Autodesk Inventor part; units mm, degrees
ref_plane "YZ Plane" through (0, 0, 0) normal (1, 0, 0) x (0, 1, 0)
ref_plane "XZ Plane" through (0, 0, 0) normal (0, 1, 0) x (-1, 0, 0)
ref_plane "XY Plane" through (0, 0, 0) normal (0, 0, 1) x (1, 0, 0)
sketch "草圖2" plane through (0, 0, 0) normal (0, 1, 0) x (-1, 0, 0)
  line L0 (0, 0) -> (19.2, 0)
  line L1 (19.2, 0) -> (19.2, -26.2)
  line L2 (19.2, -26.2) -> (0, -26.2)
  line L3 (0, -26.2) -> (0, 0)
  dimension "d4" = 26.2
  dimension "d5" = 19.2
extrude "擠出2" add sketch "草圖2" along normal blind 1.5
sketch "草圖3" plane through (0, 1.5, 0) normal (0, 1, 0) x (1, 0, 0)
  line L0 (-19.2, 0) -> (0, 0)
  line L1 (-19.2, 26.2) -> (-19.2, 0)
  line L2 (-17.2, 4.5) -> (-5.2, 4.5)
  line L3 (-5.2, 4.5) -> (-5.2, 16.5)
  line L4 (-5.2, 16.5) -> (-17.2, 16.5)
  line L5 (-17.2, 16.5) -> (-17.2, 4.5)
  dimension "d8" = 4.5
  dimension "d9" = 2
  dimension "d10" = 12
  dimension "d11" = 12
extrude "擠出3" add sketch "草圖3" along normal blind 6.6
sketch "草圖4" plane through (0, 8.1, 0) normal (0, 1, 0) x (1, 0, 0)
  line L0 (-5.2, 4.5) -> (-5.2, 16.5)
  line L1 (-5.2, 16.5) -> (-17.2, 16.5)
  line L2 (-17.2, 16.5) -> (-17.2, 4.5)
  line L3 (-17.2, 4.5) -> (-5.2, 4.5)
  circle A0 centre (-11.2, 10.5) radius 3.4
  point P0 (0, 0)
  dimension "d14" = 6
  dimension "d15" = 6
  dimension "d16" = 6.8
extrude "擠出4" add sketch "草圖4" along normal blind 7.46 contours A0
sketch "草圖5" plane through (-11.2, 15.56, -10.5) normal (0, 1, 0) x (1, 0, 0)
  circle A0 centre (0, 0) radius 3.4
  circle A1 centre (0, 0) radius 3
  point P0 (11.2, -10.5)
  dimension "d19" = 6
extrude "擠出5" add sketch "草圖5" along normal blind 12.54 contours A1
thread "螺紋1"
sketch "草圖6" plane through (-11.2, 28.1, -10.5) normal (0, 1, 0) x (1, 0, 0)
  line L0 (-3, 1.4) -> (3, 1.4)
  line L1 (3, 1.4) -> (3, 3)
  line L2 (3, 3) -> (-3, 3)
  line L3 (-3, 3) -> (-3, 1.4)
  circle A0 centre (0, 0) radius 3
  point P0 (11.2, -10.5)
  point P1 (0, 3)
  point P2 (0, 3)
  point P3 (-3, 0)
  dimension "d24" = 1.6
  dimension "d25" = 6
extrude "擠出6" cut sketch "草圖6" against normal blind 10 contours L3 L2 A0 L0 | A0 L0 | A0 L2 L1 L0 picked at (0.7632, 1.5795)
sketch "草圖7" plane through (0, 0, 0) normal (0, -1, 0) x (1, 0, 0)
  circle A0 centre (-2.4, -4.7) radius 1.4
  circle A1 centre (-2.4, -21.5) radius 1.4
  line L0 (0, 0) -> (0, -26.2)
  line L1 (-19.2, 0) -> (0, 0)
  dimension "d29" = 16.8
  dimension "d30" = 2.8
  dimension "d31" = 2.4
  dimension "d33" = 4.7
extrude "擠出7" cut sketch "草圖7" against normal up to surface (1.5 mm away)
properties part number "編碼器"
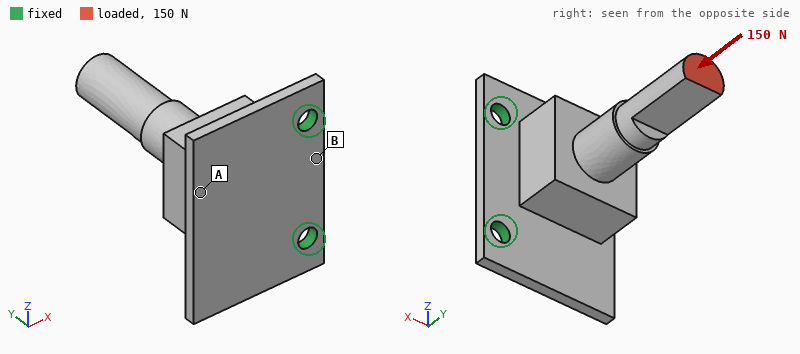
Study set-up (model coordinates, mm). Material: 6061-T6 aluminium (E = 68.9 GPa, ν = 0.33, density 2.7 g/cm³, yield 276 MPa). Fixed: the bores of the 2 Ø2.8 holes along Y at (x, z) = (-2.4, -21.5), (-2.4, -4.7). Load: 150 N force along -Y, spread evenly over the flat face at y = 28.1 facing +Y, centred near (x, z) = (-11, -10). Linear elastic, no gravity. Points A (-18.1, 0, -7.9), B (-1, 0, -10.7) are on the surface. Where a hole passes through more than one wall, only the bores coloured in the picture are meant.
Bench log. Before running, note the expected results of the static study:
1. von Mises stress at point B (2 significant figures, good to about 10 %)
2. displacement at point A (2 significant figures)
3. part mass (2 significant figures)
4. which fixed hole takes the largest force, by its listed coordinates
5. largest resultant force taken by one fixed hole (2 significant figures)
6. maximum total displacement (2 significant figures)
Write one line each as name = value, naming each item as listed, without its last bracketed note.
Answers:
von Mises stress at point B = 37 MPa
displacement at point A = 0.12 mm
part mass = 6.1 g
which fixed hole takes the largest force, by its listed coordinates = (-2.4, -4.7)
largest resultant force taken by one fixed hole = 97 N
maximum total displacement = 0.24 mm
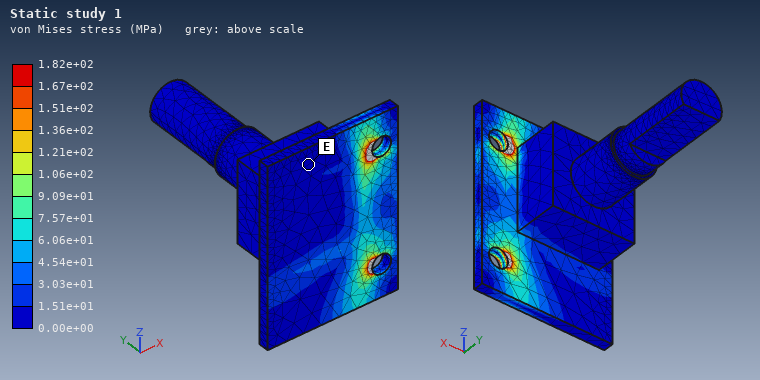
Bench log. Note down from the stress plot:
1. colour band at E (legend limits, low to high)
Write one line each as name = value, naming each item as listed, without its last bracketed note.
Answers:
colour band at E = 0.00e+00 to 1.51e+01 MPa
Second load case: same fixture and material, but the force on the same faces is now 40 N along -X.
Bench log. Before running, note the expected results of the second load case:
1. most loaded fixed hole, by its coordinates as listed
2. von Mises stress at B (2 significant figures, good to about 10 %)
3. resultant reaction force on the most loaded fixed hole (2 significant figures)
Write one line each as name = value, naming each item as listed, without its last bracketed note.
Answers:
most loaded fixed hole, by its coordinates as listed = (-2.4, -4.7)
von Mises stress at B = 46 MPa
resultant reaction force on the most loaded fixed hole = 32 N
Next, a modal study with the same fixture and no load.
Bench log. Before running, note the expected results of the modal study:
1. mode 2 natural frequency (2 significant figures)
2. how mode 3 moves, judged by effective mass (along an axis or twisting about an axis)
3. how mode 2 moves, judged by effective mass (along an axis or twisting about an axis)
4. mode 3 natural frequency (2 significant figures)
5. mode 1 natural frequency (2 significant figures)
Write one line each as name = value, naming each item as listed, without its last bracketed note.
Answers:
mode 2 natural frequency = 5700 Hz
how mode 3 moves, judged by effective mass = along Y
how mode 2 moves, judged by effective mass = along Z
mode 3 natural frequency = 12 kHz
mode 1 natural frequency = 1900 Hz
